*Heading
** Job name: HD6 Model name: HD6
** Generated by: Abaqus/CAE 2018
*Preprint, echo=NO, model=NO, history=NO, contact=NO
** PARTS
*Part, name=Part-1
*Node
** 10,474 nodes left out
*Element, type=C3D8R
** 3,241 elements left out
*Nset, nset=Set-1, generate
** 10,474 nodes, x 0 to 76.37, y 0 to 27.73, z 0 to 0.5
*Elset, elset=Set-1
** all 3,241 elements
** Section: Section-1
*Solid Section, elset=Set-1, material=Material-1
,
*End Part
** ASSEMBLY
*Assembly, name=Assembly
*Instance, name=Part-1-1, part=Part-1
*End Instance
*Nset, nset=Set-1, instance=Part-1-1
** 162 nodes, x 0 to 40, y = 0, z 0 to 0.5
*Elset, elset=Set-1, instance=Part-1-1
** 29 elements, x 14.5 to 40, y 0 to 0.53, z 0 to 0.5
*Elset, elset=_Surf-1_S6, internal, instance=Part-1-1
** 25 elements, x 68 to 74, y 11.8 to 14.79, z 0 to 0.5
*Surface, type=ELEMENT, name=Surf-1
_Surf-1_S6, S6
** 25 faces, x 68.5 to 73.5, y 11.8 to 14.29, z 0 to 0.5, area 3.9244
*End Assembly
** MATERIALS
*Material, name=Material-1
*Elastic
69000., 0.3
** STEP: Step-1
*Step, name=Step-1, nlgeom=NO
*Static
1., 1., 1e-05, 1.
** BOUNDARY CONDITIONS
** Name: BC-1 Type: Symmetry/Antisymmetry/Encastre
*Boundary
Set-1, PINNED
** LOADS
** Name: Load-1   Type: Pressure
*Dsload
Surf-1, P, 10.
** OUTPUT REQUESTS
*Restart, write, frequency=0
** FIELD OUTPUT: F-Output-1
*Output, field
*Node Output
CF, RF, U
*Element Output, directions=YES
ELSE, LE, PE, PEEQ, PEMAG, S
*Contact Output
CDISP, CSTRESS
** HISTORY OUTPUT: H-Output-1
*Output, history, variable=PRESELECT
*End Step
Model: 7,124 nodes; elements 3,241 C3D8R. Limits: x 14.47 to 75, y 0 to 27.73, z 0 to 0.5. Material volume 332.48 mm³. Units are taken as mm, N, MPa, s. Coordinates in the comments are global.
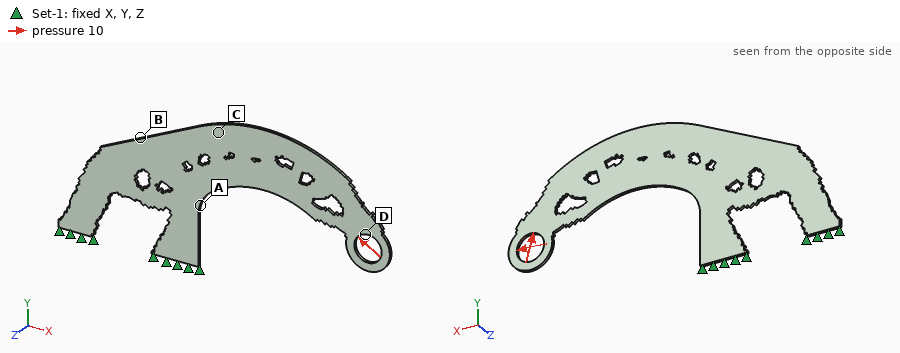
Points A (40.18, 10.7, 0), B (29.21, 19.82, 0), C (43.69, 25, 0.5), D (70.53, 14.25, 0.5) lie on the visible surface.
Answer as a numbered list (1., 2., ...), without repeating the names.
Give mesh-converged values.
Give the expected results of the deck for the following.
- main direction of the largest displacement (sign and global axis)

1. +Y
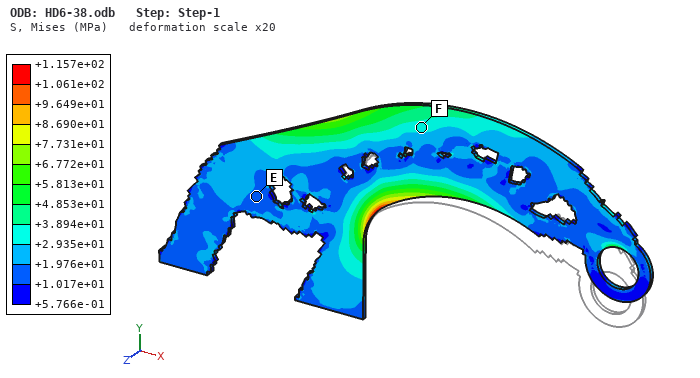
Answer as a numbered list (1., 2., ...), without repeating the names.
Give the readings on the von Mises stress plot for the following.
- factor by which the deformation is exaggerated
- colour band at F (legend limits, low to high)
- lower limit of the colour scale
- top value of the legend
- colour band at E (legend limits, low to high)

1. 20
2. +2.935e+01 to +3.894e+01 MPa
3. +5.766e-01 MPa
4. +1.157e+02 MPa
5. +1.017e+01 to +1.976e+01 MPa
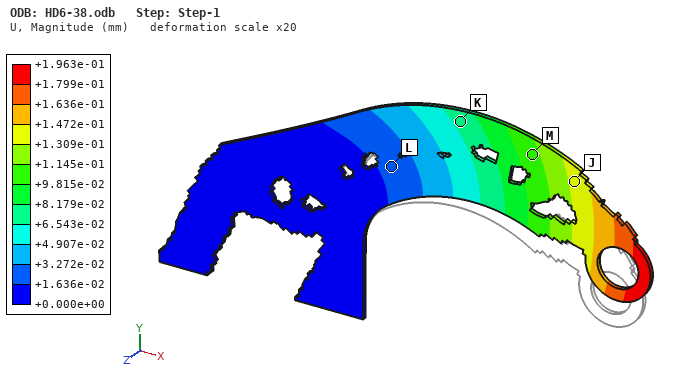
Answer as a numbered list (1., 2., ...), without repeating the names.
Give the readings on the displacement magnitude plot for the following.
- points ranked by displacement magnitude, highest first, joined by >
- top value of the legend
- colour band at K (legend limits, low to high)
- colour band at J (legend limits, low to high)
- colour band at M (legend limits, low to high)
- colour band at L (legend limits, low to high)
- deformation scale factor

1. J > M > K > L
2. +1.963e-01 mm
3. +6.543e-02 to +8.179e-02 mm
4. +1.309e-01 to +1.472e-01 mm
5. +9.815e-02 to +1.145e-01 mm
6. +1.636e-02 to +3.272e-02 mm
7. 20
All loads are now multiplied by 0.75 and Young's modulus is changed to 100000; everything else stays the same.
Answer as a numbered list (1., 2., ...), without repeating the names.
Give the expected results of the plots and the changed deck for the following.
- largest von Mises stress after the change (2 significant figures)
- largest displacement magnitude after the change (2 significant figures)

1. 87 MPa
2. 0.10 mm
